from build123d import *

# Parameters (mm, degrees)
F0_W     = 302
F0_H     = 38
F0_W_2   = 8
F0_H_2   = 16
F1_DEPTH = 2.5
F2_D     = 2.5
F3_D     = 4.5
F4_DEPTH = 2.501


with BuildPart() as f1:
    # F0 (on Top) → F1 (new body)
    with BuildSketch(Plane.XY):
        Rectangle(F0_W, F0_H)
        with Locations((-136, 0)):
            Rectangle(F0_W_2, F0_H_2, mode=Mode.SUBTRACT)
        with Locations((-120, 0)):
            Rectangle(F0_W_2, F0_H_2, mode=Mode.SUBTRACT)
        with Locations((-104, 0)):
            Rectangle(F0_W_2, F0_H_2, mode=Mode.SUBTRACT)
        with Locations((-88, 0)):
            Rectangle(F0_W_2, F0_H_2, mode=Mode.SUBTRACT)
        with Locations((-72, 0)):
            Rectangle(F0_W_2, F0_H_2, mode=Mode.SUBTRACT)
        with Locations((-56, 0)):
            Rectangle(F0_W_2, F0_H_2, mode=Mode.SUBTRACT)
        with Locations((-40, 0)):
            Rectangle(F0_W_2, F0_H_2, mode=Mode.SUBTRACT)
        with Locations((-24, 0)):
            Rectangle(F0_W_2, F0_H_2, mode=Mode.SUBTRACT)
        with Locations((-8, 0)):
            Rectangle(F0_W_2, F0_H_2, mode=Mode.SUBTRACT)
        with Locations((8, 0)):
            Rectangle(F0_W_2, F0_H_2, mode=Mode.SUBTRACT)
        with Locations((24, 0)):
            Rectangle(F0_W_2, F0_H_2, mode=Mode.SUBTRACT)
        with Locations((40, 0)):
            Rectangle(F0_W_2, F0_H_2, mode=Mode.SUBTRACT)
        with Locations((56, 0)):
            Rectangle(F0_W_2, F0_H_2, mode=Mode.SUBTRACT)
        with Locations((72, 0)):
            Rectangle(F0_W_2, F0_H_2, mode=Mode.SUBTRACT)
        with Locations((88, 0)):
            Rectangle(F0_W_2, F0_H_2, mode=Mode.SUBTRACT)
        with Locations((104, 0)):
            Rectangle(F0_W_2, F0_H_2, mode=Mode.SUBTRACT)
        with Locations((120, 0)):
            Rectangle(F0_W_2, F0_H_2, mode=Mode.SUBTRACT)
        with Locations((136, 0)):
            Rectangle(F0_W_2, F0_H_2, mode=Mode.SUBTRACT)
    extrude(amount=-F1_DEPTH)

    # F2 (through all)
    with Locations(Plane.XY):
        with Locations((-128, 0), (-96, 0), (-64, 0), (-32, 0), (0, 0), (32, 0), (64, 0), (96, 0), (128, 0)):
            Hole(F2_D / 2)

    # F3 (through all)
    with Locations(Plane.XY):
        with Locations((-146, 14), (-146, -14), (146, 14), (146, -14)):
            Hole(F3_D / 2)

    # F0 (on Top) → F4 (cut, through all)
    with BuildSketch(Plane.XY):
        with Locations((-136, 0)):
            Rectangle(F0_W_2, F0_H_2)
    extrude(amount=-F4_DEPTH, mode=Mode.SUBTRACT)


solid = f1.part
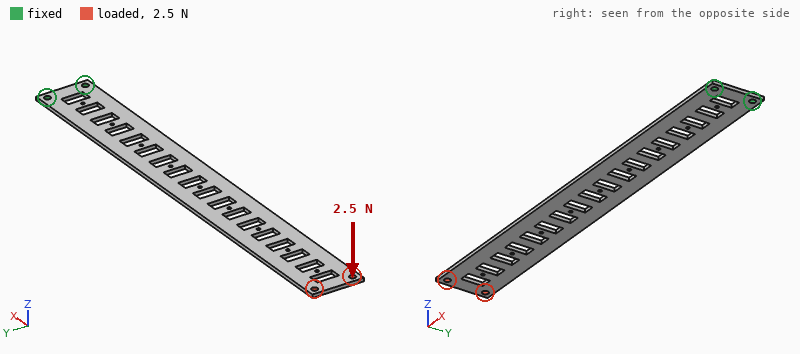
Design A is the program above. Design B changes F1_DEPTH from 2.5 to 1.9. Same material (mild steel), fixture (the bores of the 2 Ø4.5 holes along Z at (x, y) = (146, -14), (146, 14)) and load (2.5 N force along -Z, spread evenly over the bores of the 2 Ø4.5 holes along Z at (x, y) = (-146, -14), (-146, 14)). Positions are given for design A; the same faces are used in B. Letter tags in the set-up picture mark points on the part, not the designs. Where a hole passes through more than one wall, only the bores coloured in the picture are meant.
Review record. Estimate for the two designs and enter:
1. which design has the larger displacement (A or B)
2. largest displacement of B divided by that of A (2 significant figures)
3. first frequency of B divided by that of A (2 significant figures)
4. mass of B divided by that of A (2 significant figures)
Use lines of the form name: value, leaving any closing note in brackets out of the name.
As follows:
which design has the larger displacement: B
largest displacement of B divided by that of A: 2.3
first frequency of B divided by that of A: 0.76
mass of B divided by that of A: 0.76
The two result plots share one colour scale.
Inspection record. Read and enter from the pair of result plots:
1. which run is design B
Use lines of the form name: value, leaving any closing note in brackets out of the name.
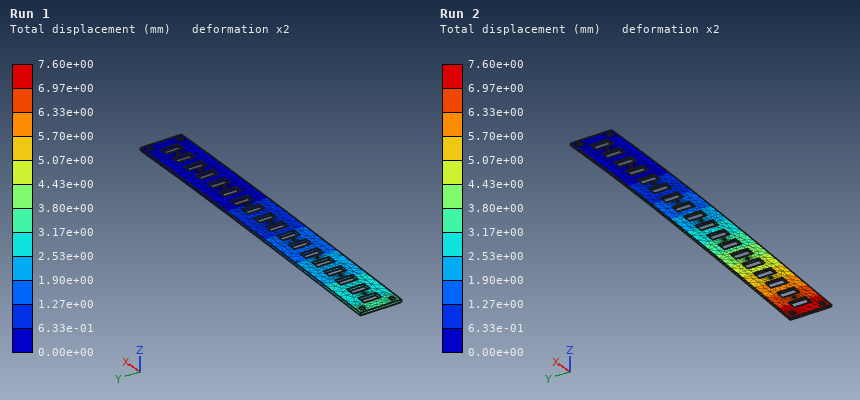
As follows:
which run is design B: Run 2
